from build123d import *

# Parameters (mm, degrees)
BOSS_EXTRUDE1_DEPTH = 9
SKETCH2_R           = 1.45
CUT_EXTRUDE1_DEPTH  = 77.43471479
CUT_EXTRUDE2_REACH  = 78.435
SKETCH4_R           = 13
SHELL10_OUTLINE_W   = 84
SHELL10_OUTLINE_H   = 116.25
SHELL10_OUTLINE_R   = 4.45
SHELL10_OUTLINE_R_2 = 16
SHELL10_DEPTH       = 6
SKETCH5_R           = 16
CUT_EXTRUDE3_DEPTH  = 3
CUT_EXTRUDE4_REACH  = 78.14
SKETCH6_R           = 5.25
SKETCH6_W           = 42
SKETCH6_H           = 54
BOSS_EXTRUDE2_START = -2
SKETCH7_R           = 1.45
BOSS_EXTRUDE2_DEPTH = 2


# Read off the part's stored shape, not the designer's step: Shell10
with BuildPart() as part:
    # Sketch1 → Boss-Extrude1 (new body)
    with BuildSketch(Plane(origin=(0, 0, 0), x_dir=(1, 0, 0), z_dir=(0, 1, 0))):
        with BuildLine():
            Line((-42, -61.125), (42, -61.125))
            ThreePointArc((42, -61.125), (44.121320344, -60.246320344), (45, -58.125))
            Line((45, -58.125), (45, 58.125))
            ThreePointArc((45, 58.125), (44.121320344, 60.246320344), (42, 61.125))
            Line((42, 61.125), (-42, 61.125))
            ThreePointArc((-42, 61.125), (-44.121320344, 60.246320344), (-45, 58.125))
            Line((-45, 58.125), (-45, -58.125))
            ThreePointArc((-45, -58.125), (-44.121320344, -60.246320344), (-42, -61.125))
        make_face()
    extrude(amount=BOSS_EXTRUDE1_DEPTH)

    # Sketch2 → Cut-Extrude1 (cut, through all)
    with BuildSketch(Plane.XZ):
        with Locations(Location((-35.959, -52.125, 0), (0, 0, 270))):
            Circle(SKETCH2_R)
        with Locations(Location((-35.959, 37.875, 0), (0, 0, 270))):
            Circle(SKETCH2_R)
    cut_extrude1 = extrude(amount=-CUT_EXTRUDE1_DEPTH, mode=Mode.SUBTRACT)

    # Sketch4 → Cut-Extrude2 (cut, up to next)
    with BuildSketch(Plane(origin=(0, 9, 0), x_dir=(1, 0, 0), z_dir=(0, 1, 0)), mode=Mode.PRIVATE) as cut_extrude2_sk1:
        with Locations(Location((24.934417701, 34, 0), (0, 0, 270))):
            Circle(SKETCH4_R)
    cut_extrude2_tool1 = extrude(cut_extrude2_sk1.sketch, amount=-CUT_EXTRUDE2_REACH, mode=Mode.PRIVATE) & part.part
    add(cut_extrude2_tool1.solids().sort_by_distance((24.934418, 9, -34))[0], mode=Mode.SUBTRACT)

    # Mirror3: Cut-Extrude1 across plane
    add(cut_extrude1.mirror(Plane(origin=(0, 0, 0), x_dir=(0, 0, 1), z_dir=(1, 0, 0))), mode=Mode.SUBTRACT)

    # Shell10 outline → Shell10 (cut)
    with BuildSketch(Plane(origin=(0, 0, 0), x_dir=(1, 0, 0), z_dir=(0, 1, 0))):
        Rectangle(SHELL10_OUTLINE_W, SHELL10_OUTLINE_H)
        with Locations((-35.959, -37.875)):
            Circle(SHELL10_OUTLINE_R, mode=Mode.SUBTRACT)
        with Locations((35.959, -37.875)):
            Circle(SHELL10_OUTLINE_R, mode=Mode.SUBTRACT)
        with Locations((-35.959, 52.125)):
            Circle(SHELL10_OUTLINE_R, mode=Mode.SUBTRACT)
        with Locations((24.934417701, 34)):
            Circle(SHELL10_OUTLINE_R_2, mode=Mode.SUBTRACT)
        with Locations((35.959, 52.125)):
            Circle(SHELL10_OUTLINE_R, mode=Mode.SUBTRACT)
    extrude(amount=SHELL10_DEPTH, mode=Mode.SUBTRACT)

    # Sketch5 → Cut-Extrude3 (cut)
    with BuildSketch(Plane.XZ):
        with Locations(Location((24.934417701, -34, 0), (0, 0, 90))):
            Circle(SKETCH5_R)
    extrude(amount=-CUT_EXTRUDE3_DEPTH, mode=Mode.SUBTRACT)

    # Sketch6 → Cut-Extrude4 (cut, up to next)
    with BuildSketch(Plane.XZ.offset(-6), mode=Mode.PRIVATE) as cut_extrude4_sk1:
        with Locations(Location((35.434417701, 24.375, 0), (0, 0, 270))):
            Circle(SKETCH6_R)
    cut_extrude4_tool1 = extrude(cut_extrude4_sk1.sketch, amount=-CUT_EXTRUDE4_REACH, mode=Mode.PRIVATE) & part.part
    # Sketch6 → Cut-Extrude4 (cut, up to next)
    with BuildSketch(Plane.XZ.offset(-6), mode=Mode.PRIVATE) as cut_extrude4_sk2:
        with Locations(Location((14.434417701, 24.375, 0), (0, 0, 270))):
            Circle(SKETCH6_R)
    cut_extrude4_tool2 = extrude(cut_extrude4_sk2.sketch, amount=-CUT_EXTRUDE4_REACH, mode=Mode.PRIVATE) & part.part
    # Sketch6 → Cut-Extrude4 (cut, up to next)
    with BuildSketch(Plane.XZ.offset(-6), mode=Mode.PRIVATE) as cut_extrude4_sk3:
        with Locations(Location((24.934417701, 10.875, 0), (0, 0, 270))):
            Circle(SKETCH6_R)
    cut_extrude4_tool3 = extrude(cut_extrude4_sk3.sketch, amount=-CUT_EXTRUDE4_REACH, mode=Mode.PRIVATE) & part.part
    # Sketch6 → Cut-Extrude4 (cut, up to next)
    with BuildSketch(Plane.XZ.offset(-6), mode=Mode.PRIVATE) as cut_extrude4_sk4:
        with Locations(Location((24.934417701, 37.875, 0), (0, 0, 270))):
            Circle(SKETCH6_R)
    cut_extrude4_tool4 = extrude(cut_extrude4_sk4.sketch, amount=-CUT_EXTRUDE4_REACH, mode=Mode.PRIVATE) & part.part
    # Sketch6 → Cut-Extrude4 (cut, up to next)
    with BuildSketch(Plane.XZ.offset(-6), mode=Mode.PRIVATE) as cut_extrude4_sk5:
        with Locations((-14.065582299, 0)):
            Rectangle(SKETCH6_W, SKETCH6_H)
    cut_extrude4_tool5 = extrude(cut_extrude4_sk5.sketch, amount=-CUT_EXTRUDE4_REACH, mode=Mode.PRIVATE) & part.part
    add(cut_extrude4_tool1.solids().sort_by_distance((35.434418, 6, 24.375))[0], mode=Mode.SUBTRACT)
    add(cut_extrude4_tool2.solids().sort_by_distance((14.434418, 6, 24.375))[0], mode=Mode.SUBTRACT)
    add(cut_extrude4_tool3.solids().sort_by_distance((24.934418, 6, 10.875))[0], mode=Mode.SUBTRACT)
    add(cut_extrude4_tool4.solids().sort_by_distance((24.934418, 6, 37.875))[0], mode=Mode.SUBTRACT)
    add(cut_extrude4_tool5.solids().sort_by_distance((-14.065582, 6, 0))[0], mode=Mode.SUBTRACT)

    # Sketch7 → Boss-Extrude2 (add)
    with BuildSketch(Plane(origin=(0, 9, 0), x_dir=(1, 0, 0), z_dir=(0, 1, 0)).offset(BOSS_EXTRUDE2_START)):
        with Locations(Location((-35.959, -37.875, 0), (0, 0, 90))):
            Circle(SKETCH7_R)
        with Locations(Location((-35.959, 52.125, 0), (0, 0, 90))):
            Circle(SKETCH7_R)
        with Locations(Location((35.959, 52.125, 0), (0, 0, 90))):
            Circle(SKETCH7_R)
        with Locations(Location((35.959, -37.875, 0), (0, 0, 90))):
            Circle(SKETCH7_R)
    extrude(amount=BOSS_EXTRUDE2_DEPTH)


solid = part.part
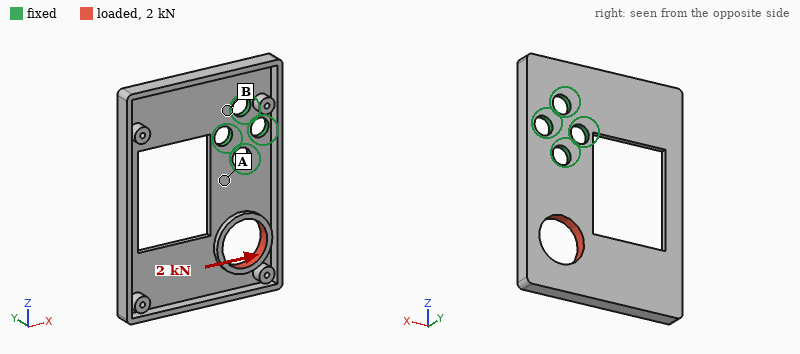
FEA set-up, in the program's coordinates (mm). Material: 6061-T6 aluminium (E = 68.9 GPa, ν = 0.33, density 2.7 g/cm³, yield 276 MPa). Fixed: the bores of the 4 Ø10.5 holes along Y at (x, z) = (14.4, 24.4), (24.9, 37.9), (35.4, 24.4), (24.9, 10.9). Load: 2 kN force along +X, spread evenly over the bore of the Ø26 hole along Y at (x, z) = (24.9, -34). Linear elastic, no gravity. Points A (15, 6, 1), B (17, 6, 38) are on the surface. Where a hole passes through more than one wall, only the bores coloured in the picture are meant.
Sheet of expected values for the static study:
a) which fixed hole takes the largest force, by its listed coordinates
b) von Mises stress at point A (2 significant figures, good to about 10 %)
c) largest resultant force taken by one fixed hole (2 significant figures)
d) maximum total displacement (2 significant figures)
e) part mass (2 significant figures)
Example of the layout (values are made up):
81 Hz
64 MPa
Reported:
(24.9, 10.9)
52 MPa
2.5 kN
0.43 mm
89 g
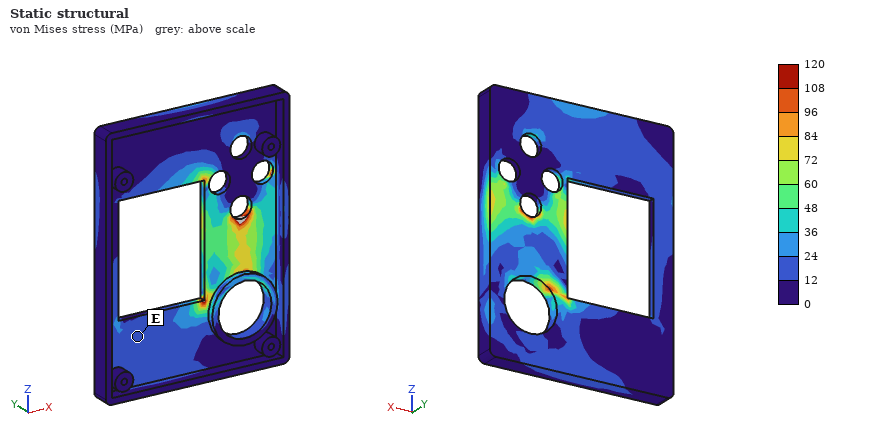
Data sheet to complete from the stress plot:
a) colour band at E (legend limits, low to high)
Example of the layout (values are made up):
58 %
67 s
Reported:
12 to 24 MPa
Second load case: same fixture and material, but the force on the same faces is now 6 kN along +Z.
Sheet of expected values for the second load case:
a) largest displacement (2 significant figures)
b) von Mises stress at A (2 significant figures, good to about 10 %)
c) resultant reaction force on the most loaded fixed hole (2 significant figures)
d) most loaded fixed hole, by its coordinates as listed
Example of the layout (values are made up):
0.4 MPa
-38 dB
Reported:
0.67 mm
86 MPa
3.1 kN
(24.9, 10.9)
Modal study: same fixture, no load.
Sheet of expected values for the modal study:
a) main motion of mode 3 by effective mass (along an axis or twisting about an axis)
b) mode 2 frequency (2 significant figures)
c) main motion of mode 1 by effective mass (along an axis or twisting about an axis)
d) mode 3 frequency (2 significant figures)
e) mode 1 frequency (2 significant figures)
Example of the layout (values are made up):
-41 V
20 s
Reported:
along Y
670 Hz
along Y
920 Hz
320 Hz
